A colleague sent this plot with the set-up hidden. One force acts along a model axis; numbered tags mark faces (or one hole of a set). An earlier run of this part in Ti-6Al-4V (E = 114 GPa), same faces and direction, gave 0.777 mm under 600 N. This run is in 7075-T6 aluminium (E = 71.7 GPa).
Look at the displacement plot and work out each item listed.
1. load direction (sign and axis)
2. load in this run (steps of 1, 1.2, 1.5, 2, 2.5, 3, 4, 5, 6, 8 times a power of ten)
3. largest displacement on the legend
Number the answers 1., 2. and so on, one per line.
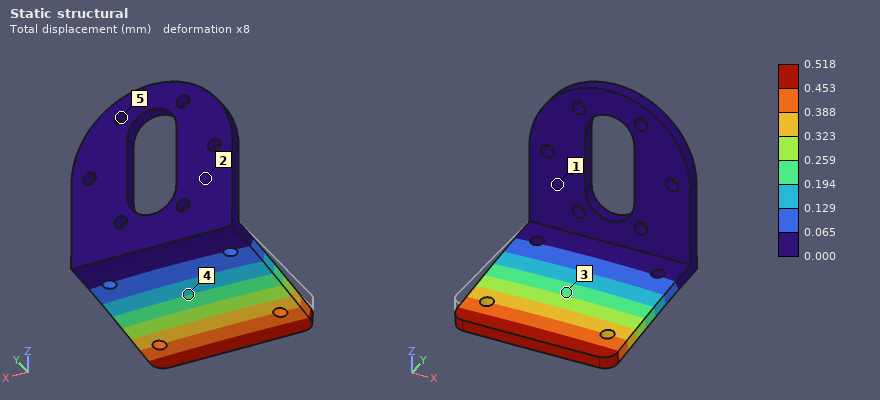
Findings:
1. -Z
2. 250 N
3. 0.518 mm
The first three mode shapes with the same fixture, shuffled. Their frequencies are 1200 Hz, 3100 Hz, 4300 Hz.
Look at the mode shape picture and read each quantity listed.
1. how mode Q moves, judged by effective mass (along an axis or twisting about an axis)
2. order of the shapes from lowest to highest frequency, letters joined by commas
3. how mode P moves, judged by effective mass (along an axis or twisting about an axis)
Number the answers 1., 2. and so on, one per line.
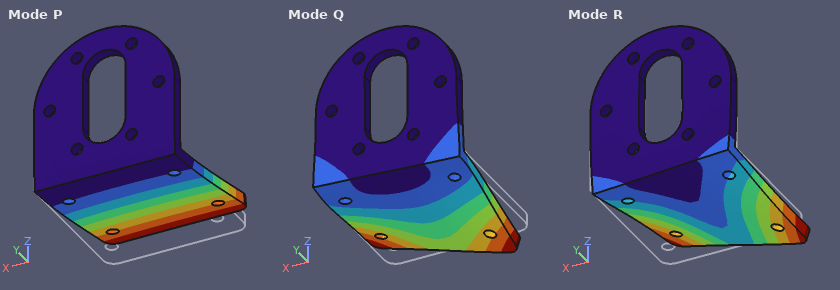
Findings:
1. along X
2. P, R, Q
3. along Z
